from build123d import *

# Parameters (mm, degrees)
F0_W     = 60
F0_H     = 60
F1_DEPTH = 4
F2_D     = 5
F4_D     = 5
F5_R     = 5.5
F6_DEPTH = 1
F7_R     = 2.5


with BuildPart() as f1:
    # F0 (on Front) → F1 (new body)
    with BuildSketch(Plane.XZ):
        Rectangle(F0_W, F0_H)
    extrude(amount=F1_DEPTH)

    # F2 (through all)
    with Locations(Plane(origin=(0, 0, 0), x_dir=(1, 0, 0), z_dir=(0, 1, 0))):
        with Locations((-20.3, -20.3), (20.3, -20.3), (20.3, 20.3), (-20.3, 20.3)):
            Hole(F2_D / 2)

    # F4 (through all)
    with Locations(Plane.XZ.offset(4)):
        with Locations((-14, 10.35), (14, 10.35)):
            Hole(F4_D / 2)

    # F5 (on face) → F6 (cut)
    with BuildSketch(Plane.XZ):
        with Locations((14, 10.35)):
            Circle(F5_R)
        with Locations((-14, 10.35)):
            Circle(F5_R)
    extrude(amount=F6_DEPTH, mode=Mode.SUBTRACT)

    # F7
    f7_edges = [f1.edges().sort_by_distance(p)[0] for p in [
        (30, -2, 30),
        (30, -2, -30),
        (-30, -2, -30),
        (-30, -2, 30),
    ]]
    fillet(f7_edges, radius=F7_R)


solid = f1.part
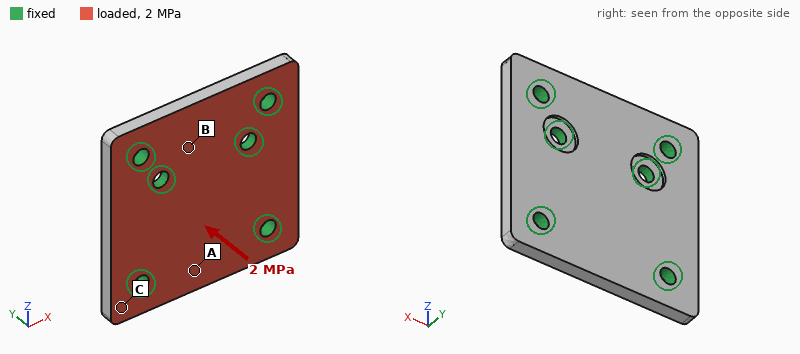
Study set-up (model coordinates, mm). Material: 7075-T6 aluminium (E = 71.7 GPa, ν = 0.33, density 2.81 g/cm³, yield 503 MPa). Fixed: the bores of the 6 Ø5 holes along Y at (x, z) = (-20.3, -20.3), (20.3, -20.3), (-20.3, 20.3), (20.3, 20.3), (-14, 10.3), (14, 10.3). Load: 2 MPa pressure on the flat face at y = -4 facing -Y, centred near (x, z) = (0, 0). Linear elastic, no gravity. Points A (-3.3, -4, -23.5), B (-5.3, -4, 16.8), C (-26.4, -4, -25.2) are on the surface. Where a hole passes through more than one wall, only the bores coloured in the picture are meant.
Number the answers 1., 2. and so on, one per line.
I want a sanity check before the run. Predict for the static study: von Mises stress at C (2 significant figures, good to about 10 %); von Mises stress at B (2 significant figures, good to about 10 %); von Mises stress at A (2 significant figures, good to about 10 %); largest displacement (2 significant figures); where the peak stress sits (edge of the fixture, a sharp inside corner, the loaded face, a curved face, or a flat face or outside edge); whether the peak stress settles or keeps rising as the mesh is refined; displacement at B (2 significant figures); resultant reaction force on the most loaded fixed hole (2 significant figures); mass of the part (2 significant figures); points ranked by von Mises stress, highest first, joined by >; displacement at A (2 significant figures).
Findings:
1. 13 MPa
2. 22 MPa
3. 41 MPa
4. 40 µm
5. edge of the fixture
6. keeps rising
7. 14 µm
8. 1.5 kN
9. 39 g
10. A > B > C
11. 34 µm
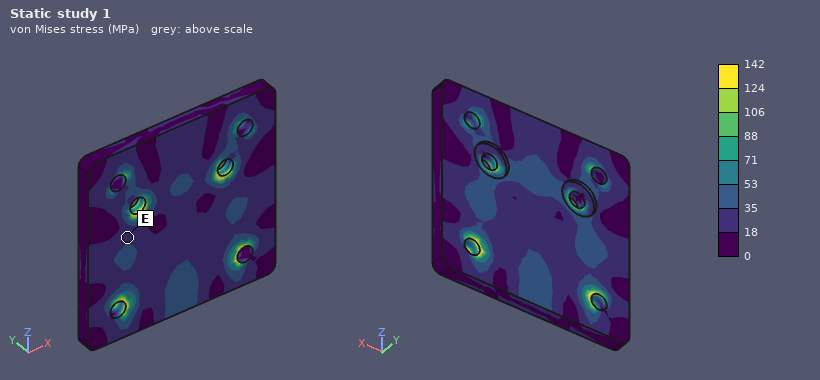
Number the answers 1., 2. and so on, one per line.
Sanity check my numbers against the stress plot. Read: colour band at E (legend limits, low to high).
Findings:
1. 18 to 35 MPa
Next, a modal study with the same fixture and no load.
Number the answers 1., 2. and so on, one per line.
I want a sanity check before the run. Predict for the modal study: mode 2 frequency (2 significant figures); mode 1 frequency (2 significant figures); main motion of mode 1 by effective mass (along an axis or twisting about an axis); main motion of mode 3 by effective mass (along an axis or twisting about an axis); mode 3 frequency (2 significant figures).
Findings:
1. 14 kHz
2. 13 kHz
3. along Y
4. along Y
5. 16 kHz
